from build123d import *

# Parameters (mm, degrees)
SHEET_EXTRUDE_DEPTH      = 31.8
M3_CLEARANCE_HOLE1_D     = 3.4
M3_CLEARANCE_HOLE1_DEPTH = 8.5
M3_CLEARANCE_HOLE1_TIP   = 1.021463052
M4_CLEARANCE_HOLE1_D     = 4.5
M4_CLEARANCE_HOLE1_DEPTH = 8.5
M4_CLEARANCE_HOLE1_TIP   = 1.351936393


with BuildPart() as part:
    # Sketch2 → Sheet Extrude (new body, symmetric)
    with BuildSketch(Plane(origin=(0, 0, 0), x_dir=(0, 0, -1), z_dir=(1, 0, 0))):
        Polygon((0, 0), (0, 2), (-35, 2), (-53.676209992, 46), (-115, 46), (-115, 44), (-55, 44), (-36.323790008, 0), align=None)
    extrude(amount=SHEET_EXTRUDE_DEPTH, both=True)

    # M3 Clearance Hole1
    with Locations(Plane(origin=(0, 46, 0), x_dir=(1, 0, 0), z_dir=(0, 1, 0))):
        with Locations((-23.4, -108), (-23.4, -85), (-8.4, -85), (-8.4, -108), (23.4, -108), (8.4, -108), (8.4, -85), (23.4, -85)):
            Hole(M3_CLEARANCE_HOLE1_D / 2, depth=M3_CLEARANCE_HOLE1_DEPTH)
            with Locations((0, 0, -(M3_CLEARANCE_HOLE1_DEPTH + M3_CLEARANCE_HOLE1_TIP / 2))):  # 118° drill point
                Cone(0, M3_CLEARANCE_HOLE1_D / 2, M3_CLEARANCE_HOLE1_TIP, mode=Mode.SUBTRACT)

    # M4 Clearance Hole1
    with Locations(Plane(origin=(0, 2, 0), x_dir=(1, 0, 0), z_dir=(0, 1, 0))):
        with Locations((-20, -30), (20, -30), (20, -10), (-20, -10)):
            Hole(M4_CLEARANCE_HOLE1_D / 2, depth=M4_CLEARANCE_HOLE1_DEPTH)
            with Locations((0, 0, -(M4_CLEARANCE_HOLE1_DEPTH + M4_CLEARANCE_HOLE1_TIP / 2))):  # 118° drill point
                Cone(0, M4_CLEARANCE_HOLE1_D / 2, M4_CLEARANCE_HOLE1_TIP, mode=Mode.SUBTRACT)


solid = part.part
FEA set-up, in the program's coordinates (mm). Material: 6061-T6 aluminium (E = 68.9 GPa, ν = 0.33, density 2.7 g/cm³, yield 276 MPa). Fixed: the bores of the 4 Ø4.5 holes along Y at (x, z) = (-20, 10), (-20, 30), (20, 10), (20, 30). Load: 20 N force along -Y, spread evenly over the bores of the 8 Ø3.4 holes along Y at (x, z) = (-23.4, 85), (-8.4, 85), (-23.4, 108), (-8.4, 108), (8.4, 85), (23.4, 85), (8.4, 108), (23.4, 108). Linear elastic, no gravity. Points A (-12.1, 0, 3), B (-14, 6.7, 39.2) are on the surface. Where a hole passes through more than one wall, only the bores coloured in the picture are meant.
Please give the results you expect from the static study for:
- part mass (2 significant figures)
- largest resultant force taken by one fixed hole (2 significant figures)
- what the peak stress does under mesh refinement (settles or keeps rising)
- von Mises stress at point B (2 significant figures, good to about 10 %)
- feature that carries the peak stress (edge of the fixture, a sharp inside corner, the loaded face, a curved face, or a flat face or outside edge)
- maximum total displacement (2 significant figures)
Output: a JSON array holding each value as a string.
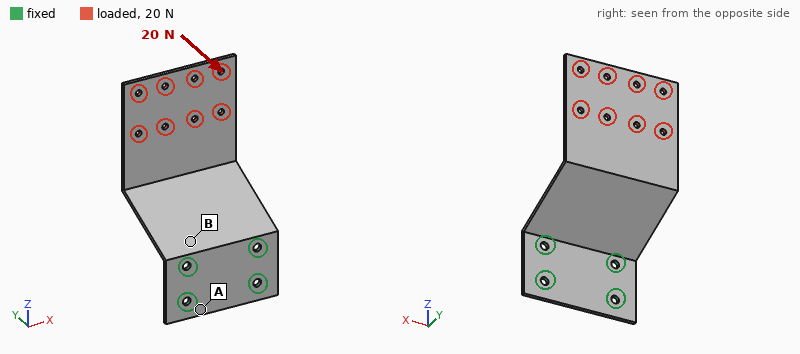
["49 g", "21 N", "keeps rising", "24 MPa", "edge of the fixture", "1.6 mm"]
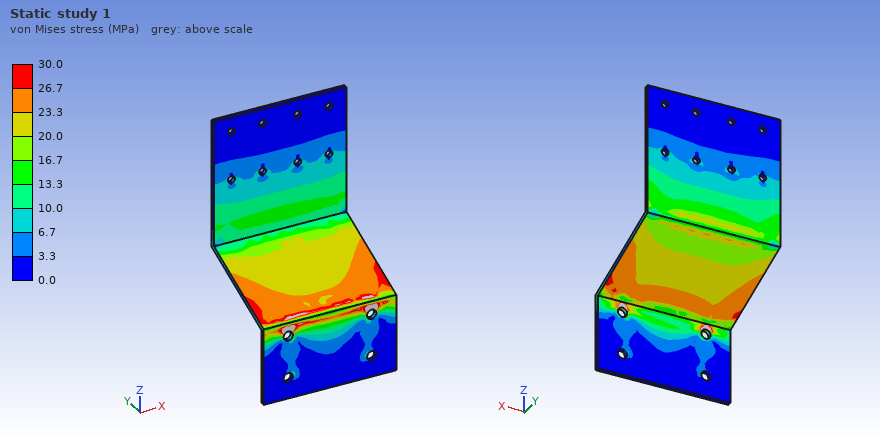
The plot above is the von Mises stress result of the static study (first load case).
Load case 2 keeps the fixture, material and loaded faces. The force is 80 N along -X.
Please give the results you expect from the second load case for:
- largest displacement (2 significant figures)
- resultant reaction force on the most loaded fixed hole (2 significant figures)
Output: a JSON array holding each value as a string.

["1.3 mm", "130 N"]
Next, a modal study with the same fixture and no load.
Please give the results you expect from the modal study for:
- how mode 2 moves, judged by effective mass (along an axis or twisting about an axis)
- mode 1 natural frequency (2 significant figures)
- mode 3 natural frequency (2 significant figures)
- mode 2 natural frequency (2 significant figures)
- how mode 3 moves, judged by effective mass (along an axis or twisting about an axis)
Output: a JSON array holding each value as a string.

["along X", "160 Hz", "570 Hz", "350 Hz", "along Z"]
